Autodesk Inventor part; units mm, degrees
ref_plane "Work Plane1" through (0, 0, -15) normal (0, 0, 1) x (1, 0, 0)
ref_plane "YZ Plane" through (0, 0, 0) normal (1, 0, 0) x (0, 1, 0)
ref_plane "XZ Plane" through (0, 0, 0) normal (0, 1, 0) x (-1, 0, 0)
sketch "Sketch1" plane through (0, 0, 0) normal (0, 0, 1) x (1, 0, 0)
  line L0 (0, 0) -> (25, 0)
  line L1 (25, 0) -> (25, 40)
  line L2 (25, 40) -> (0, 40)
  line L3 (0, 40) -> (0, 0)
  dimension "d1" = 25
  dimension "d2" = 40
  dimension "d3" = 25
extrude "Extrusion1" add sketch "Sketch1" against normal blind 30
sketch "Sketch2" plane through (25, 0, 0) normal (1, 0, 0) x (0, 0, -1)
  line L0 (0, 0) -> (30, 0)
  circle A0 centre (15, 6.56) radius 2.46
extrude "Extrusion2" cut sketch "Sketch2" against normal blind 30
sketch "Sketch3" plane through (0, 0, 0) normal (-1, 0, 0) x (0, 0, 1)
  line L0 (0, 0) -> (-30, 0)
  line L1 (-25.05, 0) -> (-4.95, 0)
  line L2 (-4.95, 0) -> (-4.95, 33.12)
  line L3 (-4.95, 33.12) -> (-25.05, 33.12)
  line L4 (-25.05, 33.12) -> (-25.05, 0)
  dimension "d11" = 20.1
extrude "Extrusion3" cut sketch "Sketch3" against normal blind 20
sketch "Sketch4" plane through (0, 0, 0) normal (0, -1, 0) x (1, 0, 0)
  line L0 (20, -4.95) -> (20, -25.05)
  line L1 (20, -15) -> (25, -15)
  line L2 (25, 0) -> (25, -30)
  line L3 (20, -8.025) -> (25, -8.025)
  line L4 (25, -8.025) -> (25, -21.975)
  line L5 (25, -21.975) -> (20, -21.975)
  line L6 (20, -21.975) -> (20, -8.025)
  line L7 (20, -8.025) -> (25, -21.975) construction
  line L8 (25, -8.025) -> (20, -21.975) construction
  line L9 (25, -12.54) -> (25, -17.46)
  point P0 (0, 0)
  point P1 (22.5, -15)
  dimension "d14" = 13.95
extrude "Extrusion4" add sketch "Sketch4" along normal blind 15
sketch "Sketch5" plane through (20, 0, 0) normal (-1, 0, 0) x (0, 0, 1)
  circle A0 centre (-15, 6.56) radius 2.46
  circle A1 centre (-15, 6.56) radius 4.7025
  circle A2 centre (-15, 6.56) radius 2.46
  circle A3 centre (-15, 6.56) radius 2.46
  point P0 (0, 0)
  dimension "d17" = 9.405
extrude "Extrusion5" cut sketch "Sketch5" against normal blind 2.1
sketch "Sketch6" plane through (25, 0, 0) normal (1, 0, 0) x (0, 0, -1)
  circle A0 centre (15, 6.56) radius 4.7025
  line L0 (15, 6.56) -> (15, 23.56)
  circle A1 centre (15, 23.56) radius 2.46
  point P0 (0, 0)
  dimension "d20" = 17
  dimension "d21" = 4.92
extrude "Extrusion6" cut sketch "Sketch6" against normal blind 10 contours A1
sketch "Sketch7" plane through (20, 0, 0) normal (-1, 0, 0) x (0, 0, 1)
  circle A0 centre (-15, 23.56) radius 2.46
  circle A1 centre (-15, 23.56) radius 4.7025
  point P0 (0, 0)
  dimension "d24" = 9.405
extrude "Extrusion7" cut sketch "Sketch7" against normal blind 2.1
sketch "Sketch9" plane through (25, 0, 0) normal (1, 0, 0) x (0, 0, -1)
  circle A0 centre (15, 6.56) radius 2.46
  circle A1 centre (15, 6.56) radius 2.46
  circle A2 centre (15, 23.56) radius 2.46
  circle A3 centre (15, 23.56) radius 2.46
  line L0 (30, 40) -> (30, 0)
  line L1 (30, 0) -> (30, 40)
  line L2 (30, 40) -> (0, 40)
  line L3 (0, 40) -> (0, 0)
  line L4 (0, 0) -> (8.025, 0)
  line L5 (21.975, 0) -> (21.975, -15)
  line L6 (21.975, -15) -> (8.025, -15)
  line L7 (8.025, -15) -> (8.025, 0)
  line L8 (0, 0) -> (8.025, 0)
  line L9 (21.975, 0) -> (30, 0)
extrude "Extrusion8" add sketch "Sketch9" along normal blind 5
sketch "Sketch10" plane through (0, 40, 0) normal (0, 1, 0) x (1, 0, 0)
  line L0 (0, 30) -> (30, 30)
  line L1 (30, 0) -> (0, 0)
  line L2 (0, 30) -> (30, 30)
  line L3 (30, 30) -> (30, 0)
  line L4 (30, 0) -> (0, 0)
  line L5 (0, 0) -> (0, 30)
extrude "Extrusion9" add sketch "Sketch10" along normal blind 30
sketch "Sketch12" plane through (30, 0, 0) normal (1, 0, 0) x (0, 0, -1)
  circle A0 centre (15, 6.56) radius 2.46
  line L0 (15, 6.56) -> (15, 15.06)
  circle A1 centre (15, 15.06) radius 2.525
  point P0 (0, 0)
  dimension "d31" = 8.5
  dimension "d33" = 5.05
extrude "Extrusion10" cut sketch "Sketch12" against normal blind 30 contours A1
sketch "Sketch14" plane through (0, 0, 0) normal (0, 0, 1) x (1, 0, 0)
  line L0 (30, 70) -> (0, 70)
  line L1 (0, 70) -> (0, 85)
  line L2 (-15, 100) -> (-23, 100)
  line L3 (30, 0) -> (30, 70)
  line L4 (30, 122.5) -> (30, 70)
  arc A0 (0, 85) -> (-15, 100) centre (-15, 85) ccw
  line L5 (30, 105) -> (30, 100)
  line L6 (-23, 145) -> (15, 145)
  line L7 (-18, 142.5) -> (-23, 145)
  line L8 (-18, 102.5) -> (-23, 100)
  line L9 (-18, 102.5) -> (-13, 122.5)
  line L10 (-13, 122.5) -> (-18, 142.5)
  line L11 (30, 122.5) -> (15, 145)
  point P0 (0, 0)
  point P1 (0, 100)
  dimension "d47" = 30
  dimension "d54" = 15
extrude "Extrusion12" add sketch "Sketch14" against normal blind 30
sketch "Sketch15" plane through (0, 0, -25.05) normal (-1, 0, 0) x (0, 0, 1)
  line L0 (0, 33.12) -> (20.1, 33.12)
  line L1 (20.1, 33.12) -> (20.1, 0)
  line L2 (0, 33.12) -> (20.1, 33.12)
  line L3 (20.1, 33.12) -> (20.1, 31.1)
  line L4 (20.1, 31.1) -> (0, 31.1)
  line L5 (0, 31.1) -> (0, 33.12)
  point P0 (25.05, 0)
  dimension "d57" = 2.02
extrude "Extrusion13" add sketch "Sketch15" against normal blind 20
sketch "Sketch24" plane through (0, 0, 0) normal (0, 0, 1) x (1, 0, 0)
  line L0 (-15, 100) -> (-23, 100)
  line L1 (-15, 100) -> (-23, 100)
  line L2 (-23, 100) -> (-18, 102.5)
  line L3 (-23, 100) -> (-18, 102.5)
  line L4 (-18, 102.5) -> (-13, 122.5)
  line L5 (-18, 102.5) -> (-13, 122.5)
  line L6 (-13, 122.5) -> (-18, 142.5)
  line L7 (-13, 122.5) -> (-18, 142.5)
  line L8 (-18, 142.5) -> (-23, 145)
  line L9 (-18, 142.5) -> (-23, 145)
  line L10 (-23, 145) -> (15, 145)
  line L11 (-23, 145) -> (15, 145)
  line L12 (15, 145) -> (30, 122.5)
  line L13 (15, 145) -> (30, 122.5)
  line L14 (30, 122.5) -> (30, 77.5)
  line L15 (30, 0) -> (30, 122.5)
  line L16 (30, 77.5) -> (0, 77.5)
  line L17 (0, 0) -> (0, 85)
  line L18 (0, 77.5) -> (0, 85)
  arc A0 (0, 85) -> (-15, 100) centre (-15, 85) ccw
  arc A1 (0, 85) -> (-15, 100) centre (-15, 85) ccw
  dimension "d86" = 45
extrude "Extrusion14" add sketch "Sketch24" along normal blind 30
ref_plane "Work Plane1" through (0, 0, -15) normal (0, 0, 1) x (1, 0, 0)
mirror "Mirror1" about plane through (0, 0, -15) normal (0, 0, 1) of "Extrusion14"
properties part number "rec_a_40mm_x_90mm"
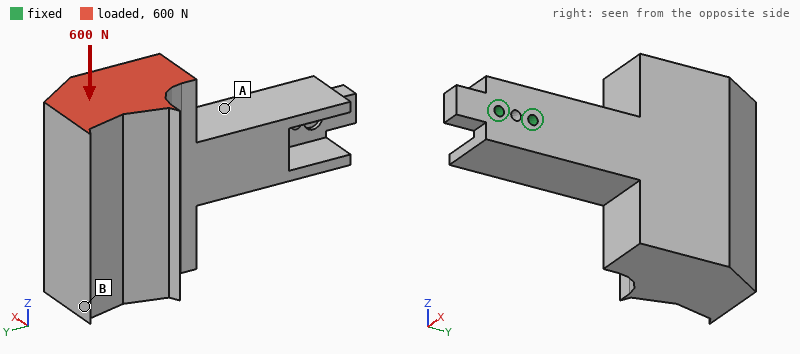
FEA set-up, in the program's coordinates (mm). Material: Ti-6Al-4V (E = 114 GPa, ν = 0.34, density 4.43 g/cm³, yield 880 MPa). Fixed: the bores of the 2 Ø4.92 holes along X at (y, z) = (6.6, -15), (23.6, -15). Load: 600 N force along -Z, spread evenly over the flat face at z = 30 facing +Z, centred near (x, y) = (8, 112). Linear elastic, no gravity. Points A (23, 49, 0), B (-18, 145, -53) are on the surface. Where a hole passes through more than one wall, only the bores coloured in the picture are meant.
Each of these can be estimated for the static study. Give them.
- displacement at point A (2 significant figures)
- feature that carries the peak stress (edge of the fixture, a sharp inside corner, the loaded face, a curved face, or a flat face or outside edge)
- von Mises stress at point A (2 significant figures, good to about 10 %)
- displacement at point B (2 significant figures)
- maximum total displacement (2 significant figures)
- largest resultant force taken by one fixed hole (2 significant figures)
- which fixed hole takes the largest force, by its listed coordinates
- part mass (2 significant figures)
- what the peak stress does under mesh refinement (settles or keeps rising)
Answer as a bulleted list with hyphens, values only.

- 17 µm
- edge of the fixture
- 9.5 MPa
- 92 µm
- 95 µm
- 2.9 kN
- (23.6, -15)
- 1.3 kg
- keeps rising
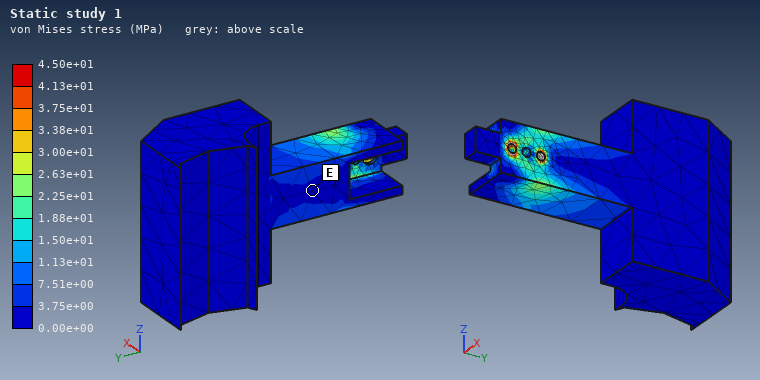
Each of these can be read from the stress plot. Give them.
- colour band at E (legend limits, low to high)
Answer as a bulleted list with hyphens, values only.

- 0.00e+00 to 3.75e+00 MPa
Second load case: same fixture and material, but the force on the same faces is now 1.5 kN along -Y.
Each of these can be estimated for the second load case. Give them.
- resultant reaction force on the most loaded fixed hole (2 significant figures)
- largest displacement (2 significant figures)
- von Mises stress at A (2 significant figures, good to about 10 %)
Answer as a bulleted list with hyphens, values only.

- 3.2 kN
- 0.15 mm
- 18 MPa
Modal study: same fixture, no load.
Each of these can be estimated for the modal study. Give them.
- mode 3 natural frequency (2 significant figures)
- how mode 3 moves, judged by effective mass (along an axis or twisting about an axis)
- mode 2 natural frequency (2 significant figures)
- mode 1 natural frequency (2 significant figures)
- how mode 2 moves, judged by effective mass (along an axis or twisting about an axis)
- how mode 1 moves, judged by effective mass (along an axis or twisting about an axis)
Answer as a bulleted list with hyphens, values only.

- 850 Hz
- twisting about Y
- 450 Hz
- 400 Hz
- along Z
- along X
